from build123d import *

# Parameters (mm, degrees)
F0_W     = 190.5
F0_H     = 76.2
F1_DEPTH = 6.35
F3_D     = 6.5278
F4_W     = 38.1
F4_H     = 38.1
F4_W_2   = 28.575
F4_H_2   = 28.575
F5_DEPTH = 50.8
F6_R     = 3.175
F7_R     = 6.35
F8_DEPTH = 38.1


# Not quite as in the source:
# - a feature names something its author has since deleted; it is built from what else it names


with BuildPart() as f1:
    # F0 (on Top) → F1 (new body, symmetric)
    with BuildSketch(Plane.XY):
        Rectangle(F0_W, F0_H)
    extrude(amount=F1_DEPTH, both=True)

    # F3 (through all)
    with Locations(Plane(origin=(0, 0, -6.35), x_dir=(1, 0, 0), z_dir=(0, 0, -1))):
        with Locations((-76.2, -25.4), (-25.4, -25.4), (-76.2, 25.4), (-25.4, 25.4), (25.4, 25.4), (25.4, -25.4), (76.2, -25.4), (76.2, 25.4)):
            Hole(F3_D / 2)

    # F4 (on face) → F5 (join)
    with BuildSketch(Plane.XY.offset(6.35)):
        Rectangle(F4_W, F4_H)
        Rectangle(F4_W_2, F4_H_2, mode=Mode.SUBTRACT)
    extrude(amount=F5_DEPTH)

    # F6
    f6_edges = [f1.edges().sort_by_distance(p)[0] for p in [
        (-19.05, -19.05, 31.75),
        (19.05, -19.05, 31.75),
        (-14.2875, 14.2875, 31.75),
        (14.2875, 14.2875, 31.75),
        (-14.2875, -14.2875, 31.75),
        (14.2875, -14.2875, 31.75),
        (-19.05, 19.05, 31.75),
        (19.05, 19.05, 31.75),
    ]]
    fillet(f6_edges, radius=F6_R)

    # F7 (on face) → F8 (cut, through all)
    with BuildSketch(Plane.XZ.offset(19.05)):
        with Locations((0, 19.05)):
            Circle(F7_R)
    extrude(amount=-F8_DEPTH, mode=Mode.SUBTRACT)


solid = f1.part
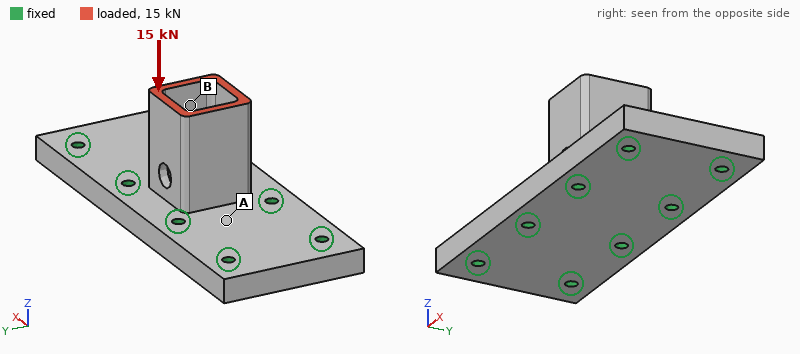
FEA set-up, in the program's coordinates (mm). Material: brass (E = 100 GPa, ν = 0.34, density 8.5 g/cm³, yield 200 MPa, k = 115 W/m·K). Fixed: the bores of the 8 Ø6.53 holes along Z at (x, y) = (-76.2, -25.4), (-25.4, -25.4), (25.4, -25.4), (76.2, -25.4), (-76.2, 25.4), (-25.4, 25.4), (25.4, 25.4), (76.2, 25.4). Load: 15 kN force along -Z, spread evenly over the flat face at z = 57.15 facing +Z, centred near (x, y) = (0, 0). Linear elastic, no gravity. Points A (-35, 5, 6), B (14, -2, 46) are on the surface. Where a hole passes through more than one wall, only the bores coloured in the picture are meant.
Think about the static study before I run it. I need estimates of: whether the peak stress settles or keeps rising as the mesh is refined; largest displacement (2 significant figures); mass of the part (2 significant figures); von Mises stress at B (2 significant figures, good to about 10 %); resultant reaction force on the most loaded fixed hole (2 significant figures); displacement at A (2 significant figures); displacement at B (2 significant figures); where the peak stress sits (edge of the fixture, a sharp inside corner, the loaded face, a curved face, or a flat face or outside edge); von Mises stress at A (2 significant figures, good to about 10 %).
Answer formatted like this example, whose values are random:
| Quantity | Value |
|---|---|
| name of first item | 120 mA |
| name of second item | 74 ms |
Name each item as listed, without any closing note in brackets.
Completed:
| Quantity | Value |
|---|---|
| whether the peak stress settles or keeps rising as the mesh is refined | keeps rising |
| largest displacement | 23 µm |
| mass of the part | 1.8 kg |
| von Mises stress at B | 25 MPa |
| resultant reaction force on the most loaded fixed hole | 3.9 kN |
| displacement at A | 4.0 µm |
| displacement at B | 19 µm |
| where the peak stress sits | edge of the fixture |
| von Mises stress at A | 9.9 MPa |
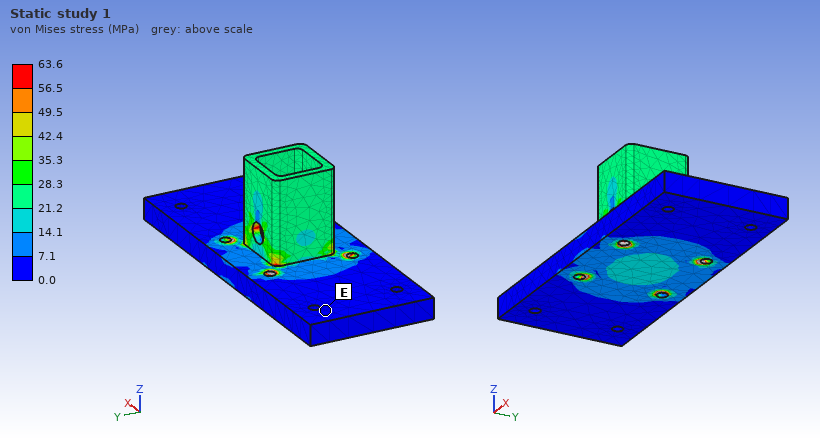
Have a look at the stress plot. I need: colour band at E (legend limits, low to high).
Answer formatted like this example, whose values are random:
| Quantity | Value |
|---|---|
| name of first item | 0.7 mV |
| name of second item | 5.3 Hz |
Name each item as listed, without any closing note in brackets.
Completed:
| Quantity | Value |
|---|---|
| colour band at E | 0.0 to 7.1 MPa |
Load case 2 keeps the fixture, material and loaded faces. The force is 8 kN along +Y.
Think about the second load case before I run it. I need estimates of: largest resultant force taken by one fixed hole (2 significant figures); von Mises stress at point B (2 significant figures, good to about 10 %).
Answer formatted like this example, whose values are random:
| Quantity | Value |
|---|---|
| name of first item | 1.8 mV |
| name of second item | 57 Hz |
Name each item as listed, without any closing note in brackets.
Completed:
| Quantity | Value |
|---|---|
| largest resultant force taken by one fixed hole | 5.4 kN |
| von Mises stress at point B | 46 MPa |
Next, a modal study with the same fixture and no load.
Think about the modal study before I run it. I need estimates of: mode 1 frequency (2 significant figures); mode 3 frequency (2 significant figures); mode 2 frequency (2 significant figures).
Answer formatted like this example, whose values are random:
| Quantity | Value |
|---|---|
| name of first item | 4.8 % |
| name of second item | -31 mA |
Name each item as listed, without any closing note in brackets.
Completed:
| Quantity | Value |
|---|---|
| mode 1 frequency | 4200 Hz |
| mode 3 frequency | 6100 Hz |
| mode 2 frequency | 4400 Hz |
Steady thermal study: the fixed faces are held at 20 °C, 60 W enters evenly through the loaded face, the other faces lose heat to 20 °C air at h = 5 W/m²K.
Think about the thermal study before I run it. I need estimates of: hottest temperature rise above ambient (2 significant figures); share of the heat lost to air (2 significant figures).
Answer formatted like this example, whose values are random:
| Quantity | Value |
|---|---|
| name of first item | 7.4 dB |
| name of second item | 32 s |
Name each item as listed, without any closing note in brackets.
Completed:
| Quantity | Value |
|---|---|
| hottest temperature rise above ambient | 51 K |
| share of the heat lost to air | 3.5 % |
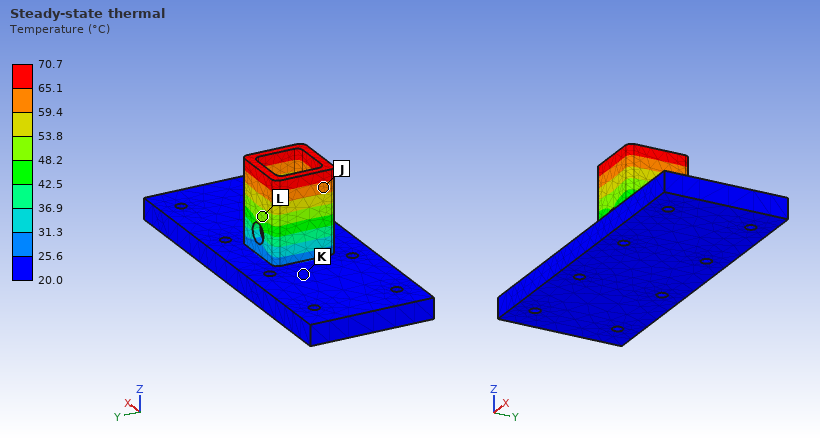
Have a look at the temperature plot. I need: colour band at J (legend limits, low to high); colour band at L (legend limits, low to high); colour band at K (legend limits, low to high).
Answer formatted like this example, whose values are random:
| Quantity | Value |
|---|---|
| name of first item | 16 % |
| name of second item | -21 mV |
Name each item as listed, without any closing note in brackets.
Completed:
| Quantity | Value |
|---|---|
| colour band at J | 59.4 to 65.1 °C |
| colour band at L | 48.2 to 53.8 °C |
| colour band at K | 20.0 to 25.6 °C |
